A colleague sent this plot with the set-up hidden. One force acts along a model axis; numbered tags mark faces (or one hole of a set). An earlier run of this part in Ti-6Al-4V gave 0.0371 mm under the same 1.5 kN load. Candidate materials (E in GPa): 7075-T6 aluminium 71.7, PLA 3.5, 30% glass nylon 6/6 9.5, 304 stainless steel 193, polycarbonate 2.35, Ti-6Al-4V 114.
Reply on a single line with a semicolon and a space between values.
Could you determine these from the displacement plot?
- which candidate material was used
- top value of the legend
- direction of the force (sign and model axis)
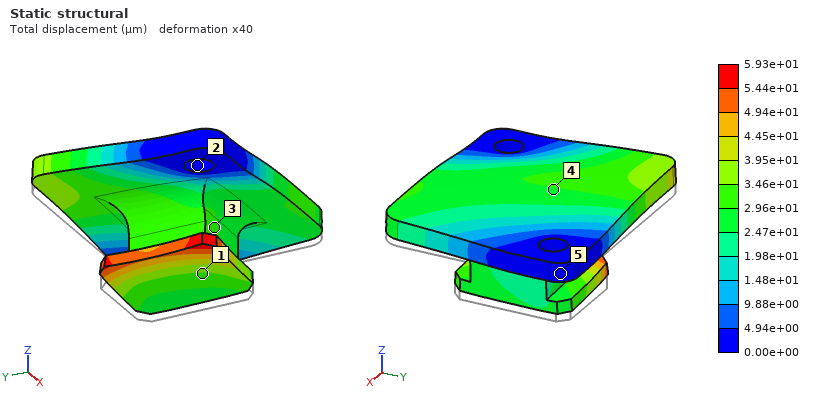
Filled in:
7075-T6 aluminium; 5.93e+01 µm; +Z
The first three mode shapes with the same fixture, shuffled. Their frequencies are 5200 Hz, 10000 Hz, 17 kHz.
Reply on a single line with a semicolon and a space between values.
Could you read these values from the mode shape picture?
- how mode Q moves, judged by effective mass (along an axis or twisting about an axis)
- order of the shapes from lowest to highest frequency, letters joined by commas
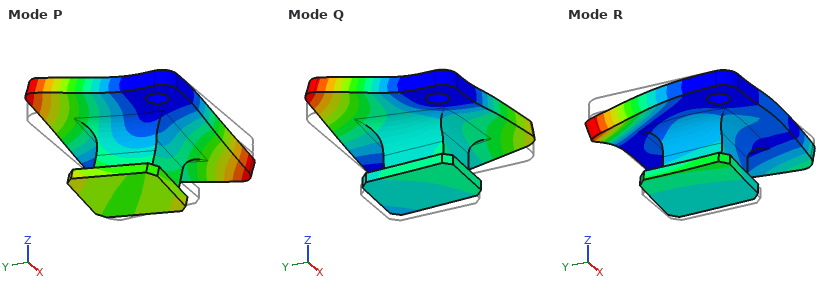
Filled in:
along Z; P, Q, R
